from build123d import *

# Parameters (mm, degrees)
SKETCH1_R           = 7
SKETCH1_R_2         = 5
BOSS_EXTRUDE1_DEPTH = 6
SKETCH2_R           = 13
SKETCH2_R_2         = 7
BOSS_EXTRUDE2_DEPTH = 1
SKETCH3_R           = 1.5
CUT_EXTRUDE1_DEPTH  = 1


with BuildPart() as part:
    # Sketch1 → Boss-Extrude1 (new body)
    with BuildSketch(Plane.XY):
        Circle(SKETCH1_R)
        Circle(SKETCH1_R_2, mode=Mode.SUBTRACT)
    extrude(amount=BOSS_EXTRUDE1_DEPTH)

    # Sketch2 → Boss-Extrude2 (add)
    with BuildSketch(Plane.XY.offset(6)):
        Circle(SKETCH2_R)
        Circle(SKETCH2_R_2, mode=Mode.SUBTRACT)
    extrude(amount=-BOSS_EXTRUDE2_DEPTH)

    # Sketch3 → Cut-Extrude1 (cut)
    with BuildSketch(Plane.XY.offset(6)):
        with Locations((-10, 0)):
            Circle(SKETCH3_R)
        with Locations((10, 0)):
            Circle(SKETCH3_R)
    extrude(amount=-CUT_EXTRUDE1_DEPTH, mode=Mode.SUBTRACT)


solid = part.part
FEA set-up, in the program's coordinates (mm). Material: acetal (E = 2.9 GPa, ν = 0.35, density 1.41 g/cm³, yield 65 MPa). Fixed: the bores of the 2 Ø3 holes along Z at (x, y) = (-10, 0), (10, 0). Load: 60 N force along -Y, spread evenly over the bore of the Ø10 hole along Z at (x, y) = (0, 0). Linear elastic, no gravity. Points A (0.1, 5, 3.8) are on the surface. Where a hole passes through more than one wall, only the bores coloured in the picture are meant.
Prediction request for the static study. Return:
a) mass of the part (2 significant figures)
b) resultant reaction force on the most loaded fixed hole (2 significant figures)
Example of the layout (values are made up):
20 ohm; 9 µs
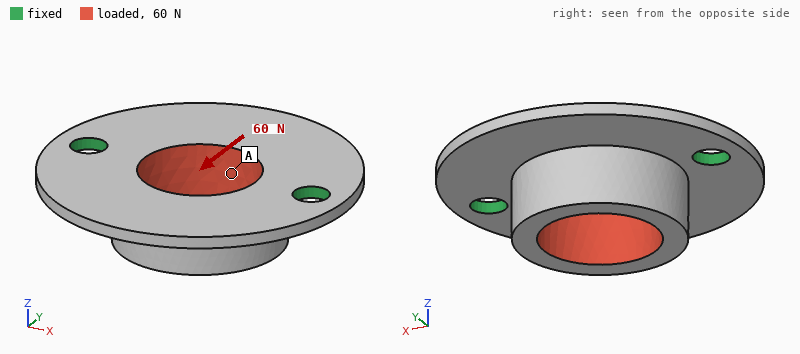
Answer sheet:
1.1 g; 30 N
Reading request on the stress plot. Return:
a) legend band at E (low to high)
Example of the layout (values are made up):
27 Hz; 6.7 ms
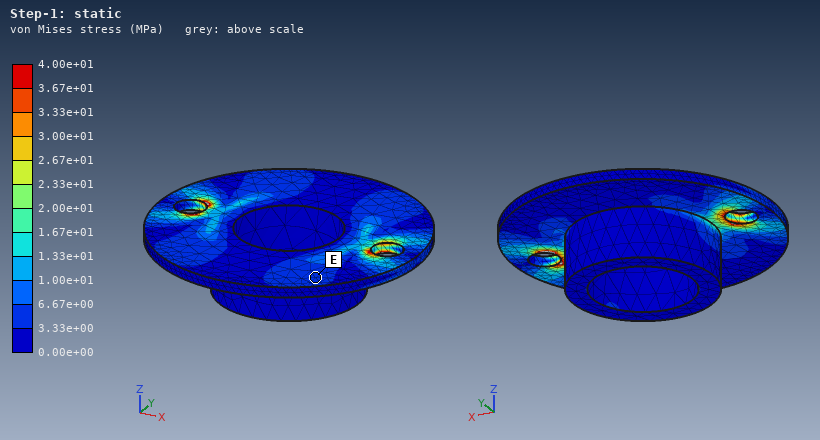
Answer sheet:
3.33e+00 to 6.67e+00 MPa
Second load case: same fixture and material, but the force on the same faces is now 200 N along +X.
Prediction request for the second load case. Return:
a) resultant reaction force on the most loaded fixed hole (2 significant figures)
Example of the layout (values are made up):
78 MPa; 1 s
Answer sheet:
100 N
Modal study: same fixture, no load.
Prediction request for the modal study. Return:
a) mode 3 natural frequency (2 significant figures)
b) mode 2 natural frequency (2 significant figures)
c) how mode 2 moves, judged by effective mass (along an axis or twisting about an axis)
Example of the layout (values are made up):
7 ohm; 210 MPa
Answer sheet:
5800 Hz; 3700 Hz; along Z
